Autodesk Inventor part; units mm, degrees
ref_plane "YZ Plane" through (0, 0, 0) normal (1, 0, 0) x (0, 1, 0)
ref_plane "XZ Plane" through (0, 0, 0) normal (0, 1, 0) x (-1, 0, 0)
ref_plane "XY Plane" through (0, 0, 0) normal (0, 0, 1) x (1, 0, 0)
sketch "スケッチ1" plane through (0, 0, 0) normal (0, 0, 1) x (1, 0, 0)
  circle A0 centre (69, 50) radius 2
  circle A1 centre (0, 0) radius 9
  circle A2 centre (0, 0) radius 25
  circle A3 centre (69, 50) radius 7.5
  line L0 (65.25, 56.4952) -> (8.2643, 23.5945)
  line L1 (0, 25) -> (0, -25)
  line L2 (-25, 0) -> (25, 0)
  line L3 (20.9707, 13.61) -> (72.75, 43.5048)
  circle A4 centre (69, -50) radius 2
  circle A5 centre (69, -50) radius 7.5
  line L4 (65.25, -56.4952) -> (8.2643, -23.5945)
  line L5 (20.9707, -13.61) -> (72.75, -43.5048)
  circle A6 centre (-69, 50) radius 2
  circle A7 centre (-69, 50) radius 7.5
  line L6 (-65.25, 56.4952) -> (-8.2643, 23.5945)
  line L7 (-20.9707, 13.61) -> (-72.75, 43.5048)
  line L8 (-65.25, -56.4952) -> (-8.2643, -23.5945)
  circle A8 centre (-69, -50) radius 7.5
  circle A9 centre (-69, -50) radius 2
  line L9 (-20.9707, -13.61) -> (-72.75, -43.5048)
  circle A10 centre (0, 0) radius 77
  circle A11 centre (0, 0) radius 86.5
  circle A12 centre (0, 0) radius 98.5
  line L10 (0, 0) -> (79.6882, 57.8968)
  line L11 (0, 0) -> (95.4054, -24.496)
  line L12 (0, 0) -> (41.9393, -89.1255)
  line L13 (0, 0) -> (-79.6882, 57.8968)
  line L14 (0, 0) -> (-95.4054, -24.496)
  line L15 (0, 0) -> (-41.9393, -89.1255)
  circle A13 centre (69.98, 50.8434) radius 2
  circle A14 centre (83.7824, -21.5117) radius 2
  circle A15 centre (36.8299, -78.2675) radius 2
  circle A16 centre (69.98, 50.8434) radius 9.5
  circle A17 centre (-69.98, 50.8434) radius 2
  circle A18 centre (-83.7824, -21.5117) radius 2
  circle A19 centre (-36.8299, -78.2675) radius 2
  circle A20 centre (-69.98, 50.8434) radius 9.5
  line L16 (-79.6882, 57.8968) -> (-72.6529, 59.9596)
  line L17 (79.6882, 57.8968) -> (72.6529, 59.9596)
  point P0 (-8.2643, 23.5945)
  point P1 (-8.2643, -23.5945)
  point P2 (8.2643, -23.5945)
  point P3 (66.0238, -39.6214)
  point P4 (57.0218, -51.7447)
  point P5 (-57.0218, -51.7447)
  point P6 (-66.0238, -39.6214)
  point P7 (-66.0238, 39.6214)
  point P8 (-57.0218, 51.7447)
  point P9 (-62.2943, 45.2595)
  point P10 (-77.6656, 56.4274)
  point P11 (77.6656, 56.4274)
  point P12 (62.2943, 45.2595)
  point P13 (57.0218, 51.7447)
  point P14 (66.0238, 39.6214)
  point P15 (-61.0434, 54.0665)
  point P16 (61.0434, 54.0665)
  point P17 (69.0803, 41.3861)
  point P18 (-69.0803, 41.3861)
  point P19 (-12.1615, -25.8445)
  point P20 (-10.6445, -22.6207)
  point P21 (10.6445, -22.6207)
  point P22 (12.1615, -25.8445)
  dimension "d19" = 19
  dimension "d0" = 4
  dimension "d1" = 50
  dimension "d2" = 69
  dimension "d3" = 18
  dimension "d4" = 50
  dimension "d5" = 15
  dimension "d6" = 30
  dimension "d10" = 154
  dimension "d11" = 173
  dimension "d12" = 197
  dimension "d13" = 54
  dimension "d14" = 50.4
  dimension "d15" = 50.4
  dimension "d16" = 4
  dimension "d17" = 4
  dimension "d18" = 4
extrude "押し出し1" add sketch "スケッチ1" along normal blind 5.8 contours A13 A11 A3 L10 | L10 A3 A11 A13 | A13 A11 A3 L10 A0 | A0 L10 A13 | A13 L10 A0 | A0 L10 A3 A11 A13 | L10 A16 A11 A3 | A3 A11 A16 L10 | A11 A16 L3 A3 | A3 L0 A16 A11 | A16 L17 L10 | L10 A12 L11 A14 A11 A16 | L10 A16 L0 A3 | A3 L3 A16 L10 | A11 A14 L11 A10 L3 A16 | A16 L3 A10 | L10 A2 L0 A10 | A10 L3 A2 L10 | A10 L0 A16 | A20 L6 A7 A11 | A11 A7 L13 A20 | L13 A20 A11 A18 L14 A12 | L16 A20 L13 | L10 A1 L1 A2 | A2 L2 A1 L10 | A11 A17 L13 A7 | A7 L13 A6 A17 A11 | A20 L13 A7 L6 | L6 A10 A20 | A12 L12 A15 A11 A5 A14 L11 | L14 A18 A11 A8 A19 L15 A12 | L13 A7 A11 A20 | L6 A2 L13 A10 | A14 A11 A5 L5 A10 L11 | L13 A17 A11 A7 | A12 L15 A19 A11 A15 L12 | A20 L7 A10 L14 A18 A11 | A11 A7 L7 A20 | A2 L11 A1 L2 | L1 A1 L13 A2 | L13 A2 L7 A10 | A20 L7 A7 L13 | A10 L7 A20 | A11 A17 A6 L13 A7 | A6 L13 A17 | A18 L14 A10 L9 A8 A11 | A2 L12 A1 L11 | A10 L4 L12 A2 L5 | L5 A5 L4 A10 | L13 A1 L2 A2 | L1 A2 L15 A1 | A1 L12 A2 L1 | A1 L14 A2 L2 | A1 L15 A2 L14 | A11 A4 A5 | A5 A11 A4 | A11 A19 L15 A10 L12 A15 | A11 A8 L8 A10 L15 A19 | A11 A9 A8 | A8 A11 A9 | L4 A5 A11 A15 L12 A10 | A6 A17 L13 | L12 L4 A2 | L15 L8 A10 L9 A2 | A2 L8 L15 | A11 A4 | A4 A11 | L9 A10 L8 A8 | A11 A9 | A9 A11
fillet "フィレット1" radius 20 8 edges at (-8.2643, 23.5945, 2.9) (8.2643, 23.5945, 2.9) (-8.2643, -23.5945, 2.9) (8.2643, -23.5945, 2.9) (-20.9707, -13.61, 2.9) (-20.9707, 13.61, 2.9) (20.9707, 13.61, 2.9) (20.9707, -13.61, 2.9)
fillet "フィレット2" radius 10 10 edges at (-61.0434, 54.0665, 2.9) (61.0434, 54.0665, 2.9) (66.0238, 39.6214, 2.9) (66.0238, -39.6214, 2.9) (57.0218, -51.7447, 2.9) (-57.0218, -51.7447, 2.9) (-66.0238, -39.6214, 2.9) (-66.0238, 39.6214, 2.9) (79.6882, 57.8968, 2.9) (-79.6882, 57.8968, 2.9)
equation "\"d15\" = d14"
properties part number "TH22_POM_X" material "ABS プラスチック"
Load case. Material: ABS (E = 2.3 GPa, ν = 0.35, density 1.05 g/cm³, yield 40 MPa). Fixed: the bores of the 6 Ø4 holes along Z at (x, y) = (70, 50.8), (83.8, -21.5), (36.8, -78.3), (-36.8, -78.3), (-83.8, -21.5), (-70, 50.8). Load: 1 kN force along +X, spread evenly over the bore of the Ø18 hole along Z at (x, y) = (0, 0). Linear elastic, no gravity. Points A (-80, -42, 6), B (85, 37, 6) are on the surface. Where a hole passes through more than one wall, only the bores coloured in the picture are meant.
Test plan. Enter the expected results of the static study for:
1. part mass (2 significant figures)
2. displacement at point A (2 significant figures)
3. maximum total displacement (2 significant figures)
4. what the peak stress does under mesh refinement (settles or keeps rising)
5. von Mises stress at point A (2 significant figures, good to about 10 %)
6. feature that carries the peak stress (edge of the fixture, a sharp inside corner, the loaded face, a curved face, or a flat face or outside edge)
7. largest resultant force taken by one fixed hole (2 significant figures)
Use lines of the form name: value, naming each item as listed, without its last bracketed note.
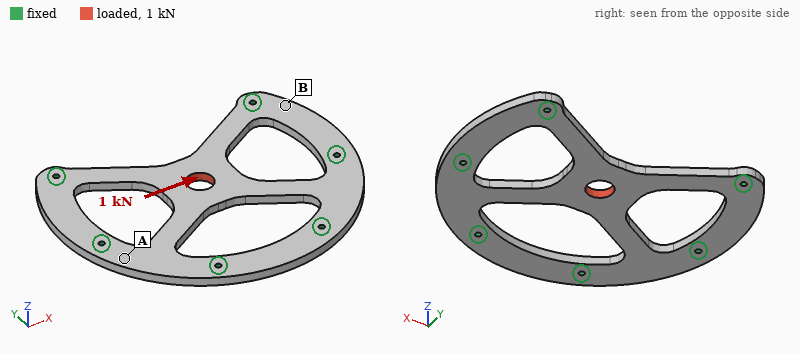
part mass: 84 g
displacement at point A: 0.053 mm
maximum total displacement: 0.18 mm
what the peak stress does under mesh refinement: keeps rising
von Mises stress at point A: 2.1 MPa
feature that carries the peak stress: edge of the fixture
largest resultant force taken by one fixed hole: 320 N
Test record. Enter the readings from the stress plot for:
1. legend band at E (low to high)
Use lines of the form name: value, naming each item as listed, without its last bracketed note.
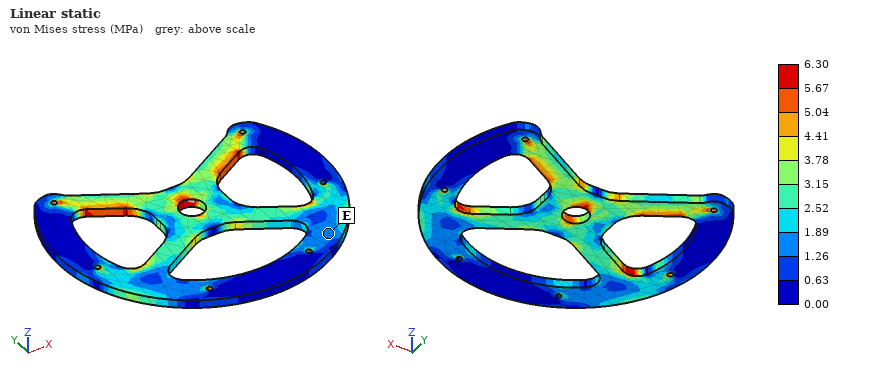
legend band at E: 1.26 to 1.89 MPa
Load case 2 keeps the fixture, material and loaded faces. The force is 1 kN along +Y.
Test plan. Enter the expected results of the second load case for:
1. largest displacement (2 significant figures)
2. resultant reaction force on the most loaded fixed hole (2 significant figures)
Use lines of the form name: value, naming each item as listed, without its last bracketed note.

largest displacement: 0.35 mm
resultant reaction force on the most loaded fixed hole: 490 N
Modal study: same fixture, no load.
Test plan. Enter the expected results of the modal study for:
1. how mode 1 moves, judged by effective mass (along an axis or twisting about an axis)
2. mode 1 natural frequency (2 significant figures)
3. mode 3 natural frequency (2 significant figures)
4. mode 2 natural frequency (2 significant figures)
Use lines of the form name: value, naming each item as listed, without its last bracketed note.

how mode 1 moves, judged by effective mass: along Z
mode 1 natural frequency: 320 Hz
mode 3 natural frequency: 830 Hz
mode 2 natural frequency: 740 Hz
